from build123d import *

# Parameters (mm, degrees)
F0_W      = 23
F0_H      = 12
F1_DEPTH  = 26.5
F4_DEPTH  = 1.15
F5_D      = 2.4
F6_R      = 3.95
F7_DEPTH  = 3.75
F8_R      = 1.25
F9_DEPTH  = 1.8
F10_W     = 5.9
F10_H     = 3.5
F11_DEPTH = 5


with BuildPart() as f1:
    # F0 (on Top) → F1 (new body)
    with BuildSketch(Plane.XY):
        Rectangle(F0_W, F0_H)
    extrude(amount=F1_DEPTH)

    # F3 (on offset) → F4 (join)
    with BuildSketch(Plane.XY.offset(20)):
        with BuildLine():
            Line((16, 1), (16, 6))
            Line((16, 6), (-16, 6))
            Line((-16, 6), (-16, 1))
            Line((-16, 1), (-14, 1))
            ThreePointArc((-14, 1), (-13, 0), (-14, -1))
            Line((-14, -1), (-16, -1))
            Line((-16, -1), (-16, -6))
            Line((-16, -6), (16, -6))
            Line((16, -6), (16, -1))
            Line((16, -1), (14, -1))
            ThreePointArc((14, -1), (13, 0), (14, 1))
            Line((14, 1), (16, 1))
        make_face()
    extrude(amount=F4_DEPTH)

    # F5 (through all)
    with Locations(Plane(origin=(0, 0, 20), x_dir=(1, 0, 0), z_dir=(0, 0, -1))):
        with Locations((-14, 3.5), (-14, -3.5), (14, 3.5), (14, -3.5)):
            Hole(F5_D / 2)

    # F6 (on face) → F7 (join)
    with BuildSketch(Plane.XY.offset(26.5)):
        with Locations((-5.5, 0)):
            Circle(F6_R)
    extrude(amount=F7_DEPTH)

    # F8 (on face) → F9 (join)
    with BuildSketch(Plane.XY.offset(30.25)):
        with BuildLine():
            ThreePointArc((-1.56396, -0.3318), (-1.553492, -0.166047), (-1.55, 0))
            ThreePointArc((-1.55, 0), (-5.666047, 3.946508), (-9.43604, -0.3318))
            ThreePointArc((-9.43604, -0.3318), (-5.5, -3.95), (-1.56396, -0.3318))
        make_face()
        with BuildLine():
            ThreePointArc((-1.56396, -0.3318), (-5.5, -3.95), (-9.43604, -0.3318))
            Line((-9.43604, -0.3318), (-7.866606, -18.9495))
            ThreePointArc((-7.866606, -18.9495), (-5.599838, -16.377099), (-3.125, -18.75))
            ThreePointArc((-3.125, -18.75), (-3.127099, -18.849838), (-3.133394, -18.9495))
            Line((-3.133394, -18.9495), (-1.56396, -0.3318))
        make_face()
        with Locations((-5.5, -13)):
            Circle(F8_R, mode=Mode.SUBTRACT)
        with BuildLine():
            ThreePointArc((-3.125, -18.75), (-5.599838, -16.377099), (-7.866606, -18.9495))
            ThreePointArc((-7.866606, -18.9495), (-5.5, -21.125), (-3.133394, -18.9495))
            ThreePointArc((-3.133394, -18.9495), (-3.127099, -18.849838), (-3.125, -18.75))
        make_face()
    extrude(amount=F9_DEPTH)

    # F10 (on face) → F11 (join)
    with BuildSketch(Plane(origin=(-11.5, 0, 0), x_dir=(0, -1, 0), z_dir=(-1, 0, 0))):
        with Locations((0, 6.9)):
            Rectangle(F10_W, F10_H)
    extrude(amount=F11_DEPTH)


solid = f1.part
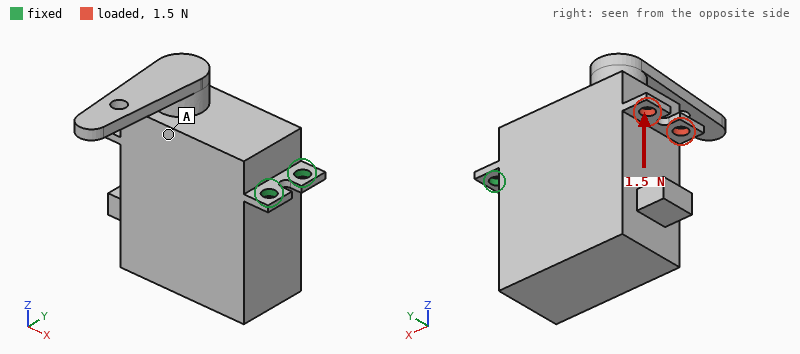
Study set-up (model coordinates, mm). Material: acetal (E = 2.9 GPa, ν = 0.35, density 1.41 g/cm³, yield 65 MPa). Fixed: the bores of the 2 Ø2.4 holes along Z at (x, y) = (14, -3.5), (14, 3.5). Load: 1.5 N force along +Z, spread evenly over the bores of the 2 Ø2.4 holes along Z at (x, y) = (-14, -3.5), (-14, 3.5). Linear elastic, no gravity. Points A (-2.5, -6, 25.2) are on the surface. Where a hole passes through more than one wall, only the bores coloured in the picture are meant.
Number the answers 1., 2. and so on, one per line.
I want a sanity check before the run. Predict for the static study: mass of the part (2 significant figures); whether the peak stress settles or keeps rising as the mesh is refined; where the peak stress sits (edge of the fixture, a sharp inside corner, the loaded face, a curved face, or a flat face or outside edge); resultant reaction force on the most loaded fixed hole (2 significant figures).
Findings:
1. 11 g
2. keeps rising
3. edge of the fixture
4. 0.75 N
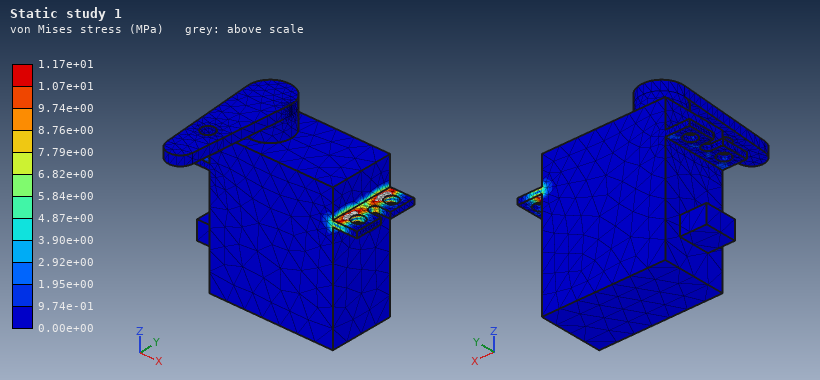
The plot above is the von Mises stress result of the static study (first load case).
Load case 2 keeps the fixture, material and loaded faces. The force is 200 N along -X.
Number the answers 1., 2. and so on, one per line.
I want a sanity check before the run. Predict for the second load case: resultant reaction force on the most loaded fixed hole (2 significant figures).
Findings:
1. 100 N
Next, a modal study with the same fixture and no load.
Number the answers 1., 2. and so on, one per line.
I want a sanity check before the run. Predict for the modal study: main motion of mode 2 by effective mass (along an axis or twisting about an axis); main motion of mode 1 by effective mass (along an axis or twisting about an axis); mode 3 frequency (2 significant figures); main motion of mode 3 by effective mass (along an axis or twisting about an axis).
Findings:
1. along Y
2. along Z
3. 1300 Hz
4. along Y
